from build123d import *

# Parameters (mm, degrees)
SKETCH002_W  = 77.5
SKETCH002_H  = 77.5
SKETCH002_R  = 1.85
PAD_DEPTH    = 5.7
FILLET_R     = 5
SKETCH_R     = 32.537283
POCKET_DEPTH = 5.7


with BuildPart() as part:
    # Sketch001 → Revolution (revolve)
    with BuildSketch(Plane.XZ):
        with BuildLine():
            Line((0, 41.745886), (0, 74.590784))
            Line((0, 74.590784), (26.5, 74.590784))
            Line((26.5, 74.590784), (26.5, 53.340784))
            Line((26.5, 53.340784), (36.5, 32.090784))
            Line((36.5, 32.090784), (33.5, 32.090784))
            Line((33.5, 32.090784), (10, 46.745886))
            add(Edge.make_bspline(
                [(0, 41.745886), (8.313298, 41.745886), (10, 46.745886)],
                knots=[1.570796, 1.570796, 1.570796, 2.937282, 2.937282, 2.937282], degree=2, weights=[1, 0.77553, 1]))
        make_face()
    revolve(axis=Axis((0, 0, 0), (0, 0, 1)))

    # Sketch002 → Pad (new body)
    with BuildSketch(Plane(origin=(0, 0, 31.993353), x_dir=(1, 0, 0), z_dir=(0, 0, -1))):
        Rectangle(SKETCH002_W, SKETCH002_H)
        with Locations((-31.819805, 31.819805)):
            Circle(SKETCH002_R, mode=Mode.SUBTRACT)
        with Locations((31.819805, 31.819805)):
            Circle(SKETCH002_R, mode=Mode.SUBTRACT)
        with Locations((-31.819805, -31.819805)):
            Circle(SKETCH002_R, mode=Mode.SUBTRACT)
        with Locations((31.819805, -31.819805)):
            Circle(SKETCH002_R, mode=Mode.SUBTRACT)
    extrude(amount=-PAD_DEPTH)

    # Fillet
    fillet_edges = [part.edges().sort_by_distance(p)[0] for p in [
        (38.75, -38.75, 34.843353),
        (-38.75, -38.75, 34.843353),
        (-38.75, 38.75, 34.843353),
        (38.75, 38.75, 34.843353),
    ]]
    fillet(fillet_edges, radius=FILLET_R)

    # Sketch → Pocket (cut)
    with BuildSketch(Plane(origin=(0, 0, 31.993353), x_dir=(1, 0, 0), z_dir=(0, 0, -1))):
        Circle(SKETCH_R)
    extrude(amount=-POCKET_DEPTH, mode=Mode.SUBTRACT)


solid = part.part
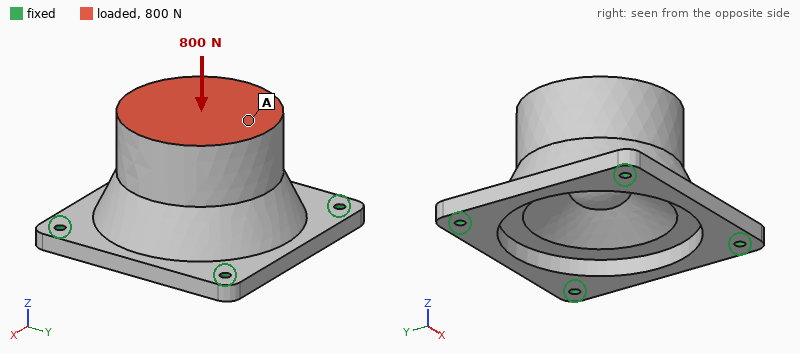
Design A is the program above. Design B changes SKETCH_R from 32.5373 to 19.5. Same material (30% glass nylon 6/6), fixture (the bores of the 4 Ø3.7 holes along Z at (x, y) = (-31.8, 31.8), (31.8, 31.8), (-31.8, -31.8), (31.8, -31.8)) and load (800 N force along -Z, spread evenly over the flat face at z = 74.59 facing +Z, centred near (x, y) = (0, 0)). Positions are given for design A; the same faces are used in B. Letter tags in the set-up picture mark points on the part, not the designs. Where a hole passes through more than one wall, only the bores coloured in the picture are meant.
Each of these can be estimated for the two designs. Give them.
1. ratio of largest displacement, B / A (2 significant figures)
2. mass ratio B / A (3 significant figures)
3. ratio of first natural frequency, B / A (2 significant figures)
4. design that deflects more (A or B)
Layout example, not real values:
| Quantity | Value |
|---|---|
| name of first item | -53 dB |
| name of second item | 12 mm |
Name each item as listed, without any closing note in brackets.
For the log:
| Quantity | Value |
|---|---|
| ratio of largest displacement, B / A | 0.85 |
| mass ratio B / A | 1.12 |
| ratio of first natural frequency, B / A | 1.1 |
| design that deflects more | A |
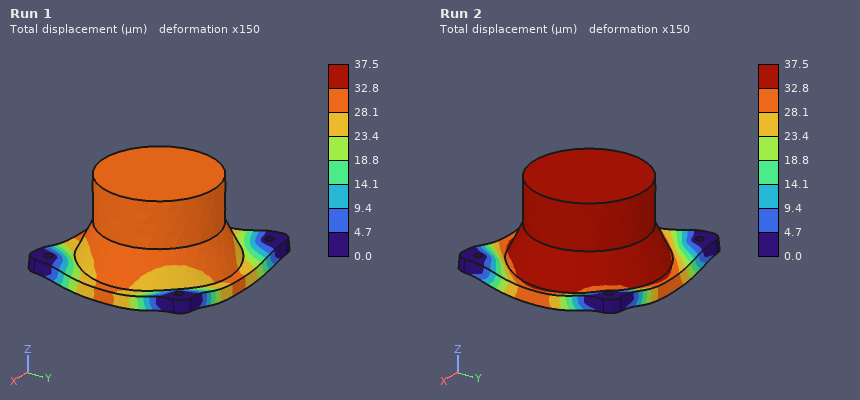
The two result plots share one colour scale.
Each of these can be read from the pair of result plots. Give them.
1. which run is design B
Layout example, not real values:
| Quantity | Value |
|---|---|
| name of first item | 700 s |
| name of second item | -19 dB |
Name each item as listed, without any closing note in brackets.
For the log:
| Quantity | Value |
|---|---|
| which run is design B | Run 1 |
